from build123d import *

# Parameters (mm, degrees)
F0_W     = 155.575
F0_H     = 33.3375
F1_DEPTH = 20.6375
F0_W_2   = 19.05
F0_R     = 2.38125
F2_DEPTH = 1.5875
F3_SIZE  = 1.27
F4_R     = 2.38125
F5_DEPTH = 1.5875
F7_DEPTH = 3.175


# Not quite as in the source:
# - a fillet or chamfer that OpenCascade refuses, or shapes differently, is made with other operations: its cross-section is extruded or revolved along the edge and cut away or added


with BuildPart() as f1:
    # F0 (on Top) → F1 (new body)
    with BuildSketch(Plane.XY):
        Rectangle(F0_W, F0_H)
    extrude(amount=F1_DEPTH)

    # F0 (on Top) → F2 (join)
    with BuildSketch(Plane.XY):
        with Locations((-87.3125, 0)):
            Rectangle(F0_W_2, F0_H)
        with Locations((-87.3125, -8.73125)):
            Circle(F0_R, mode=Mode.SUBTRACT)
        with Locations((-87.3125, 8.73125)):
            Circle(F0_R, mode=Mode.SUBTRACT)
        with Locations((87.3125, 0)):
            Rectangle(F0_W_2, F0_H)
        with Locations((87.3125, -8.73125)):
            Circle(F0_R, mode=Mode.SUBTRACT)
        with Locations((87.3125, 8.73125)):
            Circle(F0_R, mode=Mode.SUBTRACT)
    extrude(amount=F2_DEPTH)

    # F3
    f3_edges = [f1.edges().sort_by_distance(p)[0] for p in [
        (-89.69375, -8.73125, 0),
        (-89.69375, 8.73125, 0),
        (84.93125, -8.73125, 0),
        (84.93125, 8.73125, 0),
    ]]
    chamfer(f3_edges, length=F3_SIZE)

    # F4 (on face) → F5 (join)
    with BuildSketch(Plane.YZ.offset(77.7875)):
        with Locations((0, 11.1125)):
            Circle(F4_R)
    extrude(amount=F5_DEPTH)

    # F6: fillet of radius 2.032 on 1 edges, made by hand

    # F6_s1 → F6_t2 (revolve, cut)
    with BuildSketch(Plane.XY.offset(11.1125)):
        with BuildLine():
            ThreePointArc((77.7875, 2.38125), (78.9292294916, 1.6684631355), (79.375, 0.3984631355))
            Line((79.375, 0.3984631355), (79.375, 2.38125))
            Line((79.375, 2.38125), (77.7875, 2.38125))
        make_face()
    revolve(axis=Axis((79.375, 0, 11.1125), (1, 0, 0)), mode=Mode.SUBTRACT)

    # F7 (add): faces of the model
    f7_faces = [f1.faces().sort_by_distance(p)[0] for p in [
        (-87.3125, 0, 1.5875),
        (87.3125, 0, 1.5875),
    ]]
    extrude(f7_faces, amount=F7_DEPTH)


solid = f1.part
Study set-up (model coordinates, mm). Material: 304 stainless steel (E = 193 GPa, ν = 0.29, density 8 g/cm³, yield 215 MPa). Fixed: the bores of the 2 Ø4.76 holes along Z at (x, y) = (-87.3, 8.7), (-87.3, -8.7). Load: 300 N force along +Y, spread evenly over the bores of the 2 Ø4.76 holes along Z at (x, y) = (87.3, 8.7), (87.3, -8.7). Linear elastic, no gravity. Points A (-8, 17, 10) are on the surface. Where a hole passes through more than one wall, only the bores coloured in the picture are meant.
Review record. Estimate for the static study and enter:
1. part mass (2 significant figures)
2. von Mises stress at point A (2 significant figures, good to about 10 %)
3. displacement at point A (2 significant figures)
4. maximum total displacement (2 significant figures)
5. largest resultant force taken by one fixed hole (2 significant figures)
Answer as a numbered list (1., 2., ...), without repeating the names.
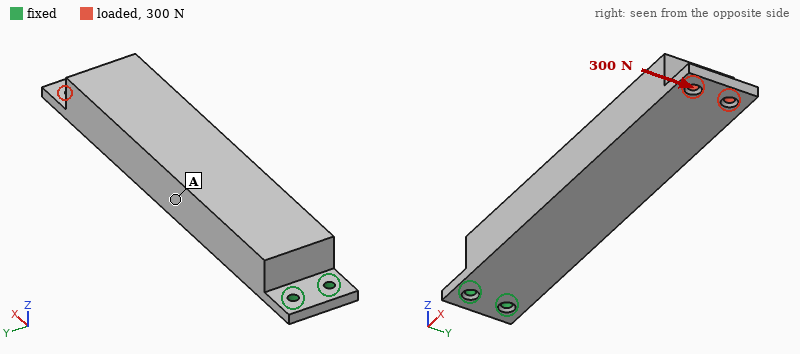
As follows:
1. 900 g
2. 7.5 MPa
3. 0.036 mm
4. 0.11 mm
5. 2.6 kN
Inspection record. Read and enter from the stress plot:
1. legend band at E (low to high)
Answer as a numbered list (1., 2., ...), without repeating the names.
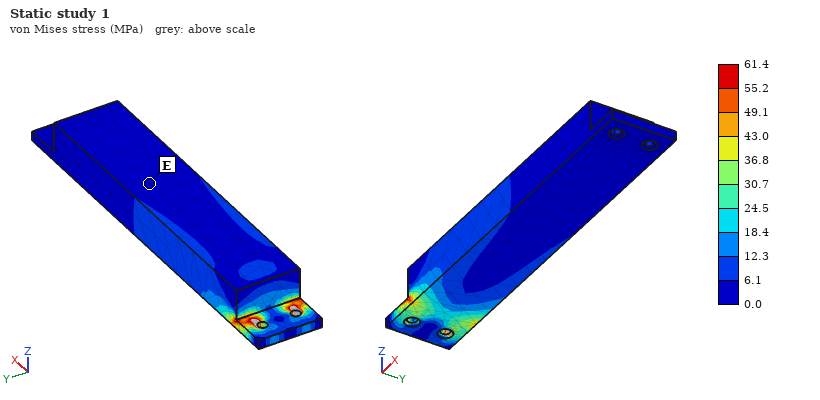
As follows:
1. 0.0 to 6.1 MPa
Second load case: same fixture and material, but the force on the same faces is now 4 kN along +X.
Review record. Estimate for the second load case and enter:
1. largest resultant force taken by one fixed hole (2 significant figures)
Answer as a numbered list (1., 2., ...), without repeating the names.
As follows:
1. 2.0 kN
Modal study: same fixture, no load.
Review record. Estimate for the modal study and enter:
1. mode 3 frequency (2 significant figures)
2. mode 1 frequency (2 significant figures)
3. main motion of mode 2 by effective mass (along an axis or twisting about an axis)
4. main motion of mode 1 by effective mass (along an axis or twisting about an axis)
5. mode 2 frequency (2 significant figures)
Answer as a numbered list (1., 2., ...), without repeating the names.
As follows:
1. 2000 Hz
2. 120 Hz
3. along Y
4. along Z
5. 560 Hz
